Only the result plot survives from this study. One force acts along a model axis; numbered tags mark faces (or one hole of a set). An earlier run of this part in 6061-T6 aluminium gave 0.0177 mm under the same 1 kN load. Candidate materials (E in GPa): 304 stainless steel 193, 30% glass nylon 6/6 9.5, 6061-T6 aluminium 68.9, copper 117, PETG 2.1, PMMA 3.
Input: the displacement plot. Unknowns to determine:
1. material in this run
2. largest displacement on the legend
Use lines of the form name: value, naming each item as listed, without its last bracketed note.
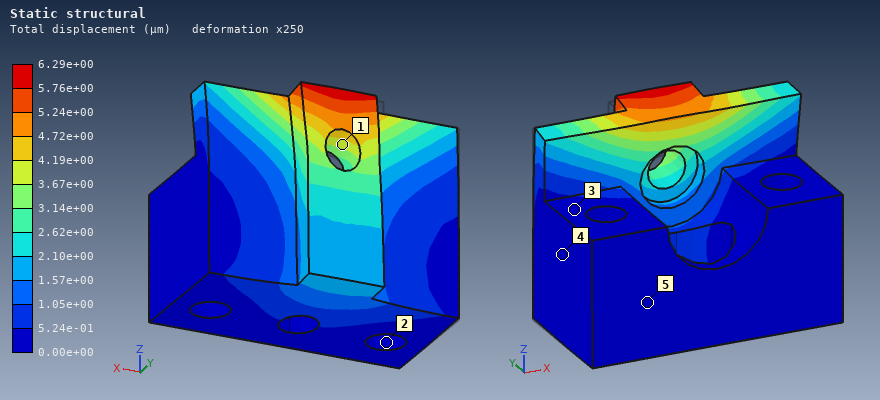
material in this run: 304 stainless steel
largest displacement on the legend: 6.29e+00 µm
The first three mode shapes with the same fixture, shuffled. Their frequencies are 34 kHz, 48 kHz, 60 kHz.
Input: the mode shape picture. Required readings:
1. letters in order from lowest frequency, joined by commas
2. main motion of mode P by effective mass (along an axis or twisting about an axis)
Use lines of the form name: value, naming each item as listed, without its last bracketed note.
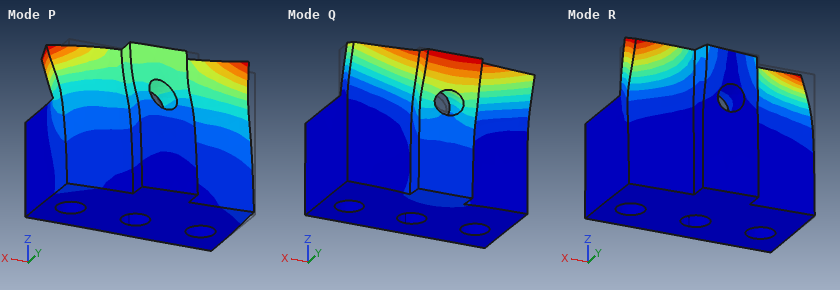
letters in order from lowest frequency, joined by commas: Q, R, P
main motion of mode P by effective mass: along X
